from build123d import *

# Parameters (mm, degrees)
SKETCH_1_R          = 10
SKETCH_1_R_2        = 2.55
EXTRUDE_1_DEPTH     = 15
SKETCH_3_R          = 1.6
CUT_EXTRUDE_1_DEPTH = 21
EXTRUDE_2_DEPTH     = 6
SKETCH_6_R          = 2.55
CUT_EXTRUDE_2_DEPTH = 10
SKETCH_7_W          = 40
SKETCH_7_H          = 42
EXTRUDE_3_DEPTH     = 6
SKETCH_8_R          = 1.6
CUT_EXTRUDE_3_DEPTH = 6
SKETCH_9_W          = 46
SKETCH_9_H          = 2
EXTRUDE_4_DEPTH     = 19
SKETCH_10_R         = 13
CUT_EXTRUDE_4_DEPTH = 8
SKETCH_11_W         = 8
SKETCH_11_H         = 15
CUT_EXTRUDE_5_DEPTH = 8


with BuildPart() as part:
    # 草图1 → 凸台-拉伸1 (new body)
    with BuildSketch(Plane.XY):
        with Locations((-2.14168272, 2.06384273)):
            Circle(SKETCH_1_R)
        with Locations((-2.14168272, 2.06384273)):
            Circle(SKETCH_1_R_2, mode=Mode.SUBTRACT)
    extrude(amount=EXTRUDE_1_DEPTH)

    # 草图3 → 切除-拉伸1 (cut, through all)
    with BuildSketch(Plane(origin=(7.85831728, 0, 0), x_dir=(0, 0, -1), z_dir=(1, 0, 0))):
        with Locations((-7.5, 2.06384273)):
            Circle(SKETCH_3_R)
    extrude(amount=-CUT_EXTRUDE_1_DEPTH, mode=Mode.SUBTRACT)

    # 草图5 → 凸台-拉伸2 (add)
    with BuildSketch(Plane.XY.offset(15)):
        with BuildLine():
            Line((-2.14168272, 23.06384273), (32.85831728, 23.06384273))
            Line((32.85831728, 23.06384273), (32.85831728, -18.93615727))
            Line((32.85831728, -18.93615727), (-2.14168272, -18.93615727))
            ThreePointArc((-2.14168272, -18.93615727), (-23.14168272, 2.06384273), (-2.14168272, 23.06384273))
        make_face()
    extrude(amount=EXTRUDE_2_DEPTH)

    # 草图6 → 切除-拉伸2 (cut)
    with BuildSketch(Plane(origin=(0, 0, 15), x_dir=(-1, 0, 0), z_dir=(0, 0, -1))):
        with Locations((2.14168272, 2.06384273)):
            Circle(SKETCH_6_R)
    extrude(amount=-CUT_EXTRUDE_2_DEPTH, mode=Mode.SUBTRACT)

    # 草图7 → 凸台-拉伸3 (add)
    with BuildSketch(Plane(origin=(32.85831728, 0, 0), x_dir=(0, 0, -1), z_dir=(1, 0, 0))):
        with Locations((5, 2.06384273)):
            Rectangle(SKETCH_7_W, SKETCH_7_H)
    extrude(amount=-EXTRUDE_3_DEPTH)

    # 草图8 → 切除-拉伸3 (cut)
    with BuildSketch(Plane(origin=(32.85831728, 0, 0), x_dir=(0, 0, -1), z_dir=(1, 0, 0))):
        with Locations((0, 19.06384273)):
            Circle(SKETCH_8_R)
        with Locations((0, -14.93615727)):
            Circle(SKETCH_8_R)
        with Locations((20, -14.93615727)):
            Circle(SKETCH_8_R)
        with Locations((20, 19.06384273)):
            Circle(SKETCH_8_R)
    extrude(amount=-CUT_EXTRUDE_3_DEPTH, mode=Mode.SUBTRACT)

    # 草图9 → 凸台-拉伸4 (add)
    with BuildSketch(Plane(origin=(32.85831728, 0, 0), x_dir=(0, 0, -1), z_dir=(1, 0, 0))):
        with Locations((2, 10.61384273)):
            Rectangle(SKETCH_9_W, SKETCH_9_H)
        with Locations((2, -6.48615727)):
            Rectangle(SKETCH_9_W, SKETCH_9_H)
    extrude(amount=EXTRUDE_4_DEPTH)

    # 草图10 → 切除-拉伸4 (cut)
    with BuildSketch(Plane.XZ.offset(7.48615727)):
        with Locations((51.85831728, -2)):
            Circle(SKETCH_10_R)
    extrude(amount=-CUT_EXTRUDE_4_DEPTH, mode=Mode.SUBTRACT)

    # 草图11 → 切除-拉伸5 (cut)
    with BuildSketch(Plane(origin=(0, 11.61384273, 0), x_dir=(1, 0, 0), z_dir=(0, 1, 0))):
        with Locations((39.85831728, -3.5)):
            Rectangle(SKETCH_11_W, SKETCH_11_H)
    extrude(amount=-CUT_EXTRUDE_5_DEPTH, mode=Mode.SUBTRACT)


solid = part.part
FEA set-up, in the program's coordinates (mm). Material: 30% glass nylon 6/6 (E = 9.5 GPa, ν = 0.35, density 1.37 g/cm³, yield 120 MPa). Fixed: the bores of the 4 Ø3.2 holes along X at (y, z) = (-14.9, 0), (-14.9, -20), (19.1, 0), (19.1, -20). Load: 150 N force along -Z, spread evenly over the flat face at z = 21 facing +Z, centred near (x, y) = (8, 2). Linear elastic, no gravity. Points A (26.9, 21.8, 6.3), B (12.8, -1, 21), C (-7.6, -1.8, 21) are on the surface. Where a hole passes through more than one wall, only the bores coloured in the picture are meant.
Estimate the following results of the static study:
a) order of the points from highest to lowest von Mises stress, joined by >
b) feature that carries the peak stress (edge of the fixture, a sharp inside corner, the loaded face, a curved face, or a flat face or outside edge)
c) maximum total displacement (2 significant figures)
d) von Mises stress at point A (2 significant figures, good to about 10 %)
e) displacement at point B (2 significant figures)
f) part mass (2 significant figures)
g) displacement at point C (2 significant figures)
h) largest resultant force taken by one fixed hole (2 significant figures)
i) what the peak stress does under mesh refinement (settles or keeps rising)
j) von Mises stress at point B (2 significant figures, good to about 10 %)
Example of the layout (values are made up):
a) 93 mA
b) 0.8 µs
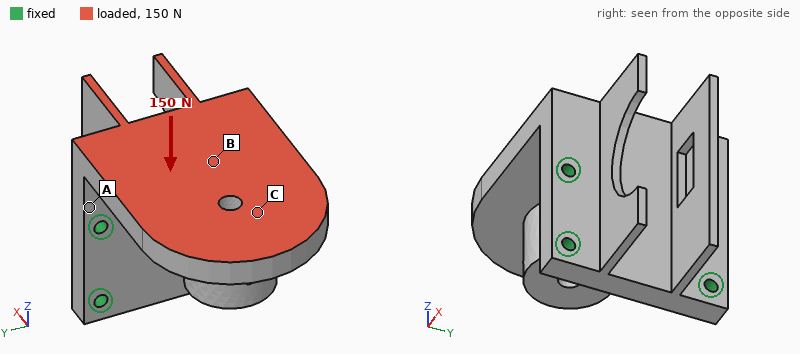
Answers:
a) A > B > C
b) edge of the fixture
c) 0.50 mm
d) 8.1 MPa
e) 0.14 mm
f) 41 g
g) 0.34 mm
h) 99 N
i) keeps rising
j) 5.0 MPa
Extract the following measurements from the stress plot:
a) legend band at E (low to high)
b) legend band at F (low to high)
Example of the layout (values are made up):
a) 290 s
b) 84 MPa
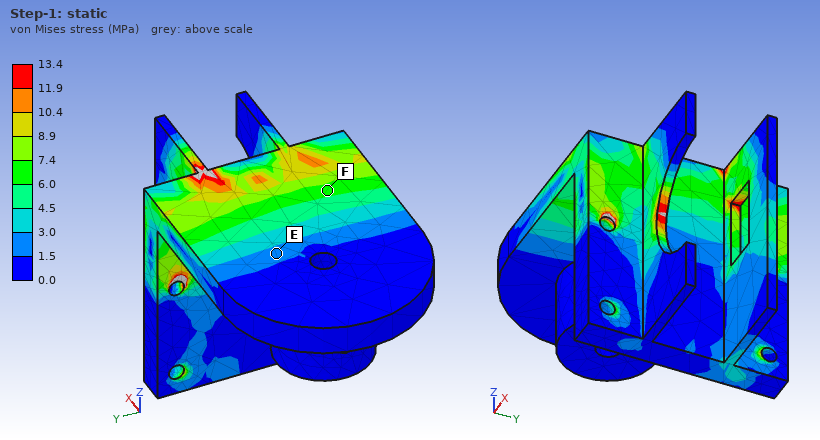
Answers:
a) 1.5 to 3.0 MPa
b) 6.0 to 7.4 MPa
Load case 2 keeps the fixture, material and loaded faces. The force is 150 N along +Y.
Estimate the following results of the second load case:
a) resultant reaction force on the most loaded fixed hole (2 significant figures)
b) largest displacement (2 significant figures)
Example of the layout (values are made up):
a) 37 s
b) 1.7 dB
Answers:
a) 150 N
b) 0.11 mm
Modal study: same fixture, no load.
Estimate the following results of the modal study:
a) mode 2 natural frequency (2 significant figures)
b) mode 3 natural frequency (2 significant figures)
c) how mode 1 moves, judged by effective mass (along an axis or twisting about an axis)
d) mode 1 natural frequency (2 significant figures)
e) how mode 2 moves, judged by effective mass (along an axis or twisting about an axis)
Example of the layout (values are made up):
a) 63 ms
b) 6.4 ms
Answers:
a) 1200 Hz
b) 1900 Hz
c) along Z
d) 670 Hz
e) along Y
